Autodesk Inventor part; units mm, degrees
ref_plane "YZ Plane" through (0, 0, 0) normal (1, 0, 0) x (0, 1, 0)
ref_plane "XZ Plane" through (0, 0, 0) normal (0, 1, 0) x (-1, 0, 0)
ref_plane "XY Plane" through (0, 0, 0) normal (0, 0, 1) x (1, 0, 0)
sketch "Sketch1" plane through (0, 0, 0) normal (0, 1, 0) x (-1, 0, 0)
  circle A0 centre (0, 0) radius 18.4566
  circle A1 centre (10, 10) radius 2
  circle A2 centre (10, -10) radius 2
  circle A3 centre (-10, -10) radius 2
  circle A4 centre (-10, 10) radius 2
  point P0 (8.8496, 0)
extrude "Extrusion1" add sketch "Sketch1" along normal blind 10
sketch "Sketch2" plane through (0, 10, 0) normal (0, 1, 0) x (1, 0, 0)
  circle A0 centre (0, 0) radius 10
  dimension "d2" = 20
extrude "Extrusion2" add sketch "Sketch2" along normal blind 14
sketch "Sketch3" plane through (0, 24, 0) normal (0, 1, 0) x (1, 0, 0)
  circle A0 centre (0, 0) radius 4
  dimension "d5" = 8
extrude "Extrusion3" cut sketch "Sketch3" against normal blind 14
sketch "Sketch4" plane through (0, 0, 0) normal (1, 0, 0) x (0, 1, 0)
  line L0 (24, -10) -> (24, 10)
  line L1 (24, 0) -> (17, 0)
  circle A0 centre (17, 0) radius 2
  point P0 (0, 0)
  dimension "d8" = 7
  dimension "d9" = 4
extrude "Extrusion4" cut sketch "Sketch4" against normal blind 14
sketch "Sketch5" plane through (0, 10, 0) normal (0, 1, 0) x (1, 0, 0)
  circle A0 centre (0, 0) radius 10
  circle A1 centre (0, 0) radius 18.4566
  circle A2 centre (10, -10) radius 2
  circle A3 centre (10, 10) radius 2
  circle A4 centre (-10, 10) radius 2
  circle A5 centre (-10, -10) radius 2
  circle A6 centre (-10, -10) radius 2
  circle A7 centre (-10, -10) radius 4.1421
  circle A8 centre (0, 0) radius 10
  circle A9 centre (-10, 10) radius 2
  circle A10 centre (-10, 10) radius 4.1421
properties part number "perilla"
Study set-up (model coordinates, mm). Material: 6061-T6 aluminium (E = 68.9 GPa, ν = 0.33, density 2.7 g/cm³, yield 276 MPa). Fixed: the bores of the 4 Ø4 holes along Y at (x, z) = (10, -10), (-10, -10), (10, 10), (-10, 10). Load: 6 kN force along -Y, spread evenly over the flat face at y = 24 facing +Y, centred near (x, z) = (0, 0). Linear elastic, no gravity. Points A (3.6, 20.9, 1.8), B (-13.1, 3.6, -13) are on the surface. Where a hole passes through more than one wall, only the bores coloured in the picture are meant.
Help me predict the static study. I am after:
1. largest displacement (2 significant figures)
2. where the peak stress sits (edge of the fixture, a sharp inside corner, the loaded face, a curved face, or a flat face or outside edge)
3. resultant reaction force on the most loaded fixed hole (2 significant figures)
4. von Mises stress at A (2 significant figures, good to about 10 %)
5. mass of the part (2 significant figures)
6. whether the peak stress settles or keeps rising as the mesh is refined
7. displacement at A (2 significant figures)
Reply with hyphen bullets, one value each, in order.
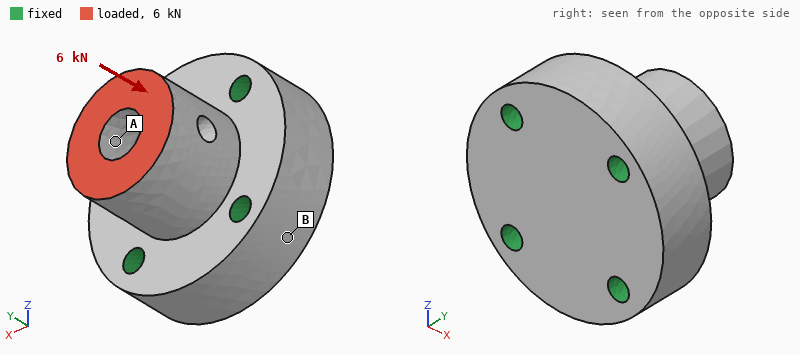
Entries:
- 10 µm
- edge of the fixture
- 1.6 kN
- 23 MPa
- 37 g
- keeps rising
- 6.9 µm
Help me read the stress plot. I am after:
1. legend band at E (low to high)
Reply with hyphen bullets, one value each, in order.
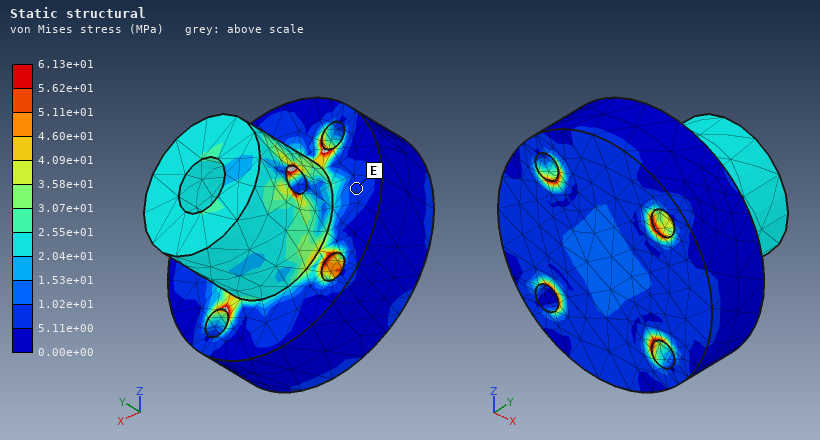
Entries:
- 5.11e+00 to 1.02e+01 MPa
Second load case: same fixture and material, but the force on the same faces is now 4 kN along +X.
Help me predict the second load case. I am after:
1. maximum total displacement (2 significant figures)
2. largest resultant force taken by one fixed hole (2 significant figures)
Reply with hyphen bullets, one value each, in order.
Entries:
- 37 µm
- 2.1 kN
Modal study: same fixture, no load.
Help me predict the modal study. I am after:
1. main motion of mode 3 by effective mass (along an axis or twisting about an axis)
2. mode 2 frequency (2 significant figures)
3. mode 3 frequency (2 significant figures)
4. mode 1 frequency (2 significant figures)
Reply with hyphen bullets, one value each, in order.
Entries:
- along Y
- 29 kHz
- 43 kHz
- 28 kHz
